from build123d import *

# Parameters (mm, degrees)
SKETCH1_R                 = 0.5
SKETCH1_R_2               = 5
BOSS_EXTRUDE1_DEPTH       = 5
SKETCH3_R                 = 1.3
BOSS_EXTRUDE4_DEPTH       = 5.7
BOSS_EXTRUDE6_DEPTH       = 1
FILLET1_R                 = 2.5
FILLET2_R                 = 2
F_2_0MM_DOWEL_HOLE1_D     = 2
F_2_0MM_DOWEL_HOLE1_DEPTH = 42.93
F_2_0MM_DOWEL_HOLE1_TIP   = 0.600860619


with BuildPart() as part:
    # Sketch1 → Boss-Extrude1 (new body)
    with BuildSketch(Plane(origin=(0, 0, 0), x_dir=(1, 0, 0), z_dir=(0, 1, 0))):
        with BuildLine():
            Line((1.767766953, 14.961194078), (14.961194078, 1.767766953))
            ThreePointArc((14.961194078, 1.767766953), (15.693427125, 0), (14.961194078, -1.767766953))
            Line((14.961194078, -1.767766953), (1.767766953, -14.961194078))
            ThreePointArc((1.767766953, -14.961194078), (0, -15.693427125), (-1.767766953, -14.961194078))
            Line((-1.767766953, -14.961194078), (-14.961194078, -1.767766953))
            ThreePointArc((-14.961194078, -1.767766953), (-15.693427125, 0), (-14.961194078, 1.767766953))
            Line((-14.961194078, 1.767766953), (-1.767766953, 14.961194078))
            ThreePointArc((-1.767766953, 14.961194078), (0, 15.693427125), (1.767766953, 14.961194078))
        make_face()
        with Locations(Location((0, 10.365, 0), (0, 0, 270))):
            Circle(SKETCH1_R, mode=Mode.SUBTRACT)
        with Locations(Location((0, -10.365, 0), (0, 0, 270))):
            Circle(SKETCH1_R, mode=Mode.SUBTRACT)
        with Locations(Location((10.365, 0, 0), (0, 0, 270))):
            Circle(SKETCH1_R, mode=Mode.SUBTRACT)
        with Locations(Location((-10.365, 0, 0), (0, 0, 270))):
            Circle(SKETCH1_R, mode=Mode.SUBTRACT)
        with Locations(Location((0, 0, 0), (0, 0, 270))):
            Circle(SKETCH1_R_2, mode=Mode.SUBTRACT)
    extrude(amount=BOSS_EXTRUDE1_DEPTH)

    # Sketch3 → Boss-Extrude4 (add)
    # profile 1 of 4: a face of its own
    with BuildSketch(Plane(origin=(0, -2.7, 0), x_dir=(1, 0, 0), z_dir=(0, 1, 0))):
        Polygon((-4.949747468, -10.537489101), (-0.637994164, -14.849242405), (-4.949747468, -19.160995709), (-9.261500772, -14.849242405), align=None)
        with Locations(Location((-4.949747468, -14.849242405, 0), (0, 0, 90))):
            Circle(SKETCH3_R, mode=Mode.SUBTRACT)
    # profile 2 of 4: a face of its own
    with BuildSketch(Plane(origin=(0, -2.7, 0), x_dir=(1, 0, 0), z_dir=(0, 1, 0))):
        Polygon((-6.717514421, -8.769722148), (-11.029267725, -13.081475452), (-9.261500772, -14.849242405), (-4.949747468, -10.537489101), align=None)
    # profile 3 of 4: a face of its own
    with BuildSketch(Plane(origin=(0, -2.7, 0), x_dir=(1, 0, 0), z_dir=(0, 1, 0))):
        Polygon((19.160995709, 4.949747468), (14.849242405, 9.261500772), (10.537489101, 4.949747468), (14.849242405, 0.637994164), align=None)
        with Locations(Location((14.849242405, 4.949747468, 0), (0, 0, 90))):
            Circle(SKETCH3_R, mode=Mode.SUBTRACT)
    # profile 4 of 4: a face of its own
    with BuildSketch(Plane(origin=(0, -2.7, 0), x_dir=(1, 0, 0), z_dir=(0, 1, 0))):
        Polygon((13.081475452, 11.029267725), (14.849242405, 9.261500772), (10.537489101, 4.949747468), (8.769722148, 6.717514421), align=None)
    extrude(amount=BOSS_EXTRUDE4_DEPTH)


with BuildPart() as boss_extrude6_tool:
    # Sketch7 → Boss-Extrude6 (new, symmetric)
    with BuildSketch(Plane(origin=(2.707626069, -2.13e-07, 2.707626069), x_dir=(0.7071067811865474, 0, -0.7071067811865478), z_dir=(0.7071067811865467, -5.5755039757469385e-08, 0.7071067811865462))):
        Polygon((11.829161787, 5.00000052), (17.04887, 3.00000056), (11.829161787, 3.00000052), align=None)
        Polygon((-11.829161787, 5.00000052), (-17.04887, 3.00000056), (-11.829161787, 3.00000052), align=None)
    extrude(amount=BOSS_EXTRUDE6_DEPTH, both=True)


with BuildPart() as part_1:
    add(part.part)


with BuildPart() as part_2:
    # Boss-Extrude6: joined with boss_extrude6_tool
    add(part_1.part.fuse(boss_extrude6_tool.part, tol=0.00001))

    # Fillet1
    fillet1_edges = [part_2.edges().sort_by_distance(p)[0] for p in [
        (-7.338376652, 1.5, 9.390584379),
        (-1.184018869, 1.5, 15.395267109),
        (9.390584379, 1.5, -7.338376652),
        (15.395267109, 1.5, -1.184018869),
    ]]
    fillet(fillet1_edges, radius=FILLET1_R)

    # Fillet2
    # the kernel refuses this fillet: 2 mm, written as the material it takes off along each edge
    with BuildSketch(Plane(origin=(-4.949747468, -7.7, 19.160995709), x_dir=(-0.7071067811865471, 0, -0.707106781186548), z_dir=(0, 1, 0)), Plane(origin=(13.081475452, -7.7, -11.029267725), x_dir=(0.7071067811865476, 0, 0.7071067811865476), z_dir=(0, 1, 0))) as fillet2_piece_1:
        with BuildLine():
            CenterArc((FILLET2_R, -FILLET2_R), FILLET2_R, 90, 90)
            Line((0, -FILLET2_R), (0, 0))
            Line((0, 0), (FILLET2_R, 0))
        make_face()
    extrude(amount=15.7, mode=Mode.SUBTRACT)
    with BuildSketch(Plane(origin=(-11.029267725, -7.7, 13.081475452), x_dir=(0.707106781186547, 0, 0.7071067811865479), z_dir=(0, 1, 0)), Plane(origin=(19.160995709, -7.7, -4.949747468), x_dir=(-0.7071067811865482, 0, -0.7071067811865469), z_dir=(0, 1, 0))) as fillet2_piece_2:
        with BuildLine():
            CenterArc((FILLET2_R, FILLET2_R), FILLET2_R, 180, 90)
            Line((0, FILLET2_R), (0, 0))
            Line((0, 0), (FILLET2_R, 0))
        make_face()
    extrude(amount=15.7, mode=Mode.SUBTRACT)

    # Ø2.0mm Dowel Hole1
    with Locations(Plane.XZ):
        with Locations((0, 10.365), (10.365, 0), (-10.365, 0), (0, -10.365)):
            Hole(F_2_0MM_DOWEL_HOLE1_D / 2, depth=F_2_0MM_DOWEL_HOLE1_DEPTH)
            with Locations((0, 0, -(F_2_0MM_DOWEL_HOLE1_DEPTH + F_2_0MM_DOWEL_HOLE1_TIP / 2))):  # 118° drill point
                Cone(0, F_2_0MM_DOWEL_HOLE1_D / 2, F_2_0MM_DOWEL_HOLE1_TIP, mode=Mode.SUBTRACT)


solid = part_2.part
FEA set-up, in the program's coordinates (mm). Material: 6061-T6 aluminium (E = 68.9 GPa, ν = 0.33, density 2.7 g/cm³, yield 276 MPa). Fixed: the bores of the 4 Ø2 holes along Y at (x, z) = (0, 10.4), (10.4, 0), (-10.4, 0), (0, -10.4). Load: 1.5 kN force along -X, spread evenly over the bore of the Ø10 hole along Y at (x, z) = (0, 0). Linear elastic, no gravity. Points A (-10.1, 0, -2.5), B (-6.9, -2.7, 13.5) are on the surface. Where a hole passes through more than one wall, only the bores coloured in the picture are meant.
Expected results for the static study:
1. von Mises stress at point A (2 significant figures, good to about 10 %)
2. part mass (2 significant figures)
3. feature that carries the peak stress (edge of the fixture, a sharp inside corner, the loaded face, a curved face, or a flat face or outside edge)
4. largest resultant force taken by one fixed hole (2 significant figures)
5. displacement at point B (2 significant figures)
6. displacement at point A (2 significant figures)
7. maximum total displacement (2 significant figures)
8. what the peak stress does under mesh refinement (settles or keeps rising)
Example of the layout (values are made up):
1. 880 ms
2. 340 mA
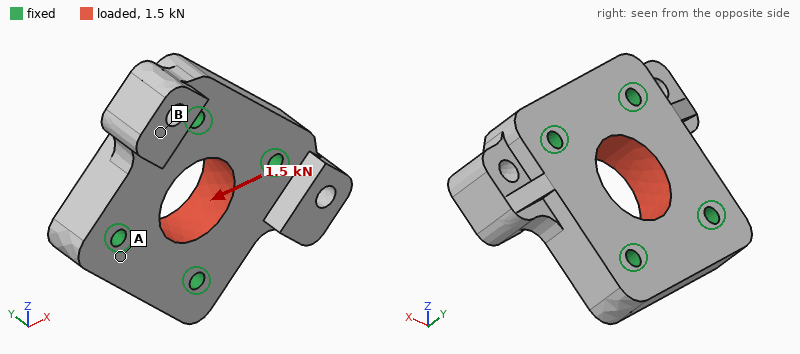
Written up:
1. 8.1 MPa
2. 7.6 g
3. edge of the fixture
4. 460 N
5. 0.64 µm
6. 0.50 µm
7. 1.7 µm
8. keeps rising
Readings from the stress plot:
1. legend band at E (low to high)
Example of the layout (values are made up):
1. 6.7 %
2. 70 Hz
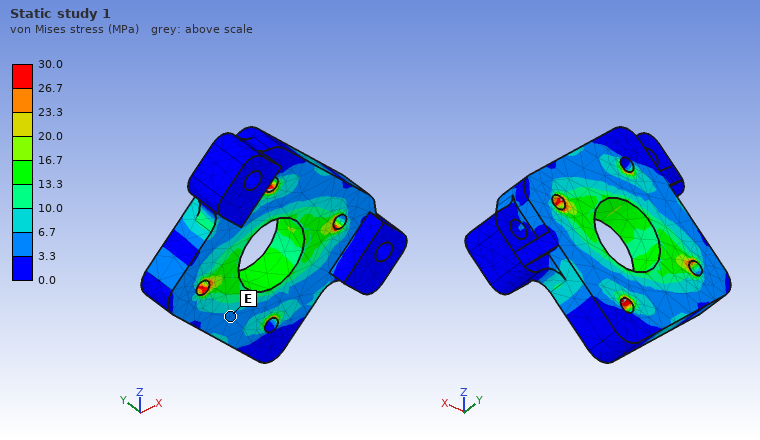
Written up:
1. 3.3 to 6.7 MPa
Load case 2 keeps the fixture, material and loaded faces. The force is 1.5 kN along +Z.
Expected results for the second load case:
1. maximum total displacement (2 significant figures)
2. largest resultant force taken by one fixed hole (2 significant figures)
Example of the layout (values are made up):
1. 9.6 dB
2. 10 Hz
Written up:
1. 1.7 µm
2. 460 N
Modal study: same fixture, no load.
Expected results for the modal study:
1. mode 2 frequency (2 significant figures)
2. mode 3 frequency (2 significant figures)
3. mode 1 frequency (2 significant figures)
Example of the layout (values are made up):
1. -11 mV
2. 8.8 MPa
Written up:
1. 31 kHz
2. 51 kHz
3. 31 kHz
